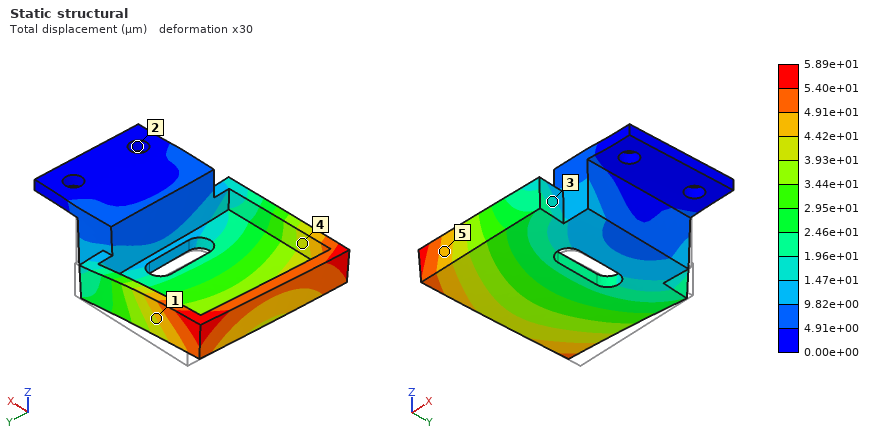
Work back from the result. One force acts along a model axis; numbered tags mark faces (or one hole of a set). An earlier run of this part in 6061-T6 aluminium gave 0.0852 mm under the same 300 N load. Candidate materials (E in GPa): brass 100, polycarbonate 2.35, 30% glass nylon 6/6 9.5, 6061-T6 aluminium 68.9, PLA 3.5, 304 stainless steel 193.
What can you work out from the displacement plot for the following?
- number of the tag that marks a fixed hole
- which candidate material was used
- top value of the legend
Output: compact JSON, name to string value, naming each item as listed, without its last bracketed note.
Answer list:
{"number of the tag that marks a fixed hole": "2", "which candidate material was used": "brass", "top value of the legend": "5.89e+01 µm"}
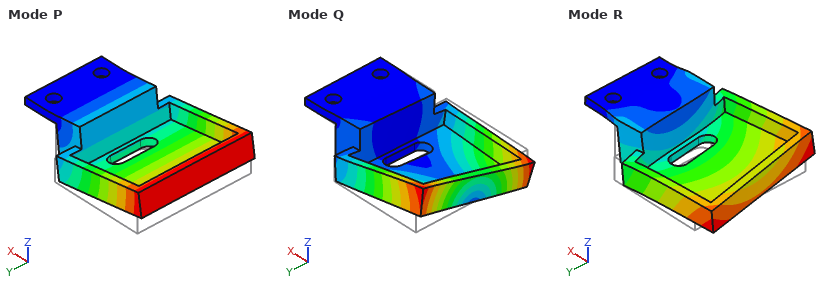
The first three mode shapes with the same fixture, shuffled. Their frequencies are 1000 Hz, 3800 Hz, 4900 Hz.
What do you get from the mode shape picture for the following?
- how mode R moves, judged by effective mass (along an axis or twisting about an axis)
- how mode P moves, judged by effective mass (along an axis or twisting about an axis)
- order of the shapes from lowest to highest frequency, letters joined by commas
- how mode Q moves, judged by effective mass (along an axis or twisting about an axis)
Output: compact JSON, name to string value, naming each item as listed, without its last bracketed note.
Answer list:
{"how mode R moves, judged by effective mass": "along Y", "how mode P moves, judged by effective mass": "along Z", "order of the shapes from lowest to highest frequency, letters joined by commas": "P, Q, R", "how mode Q moves, judged by effective mass": "twisting about X"}
